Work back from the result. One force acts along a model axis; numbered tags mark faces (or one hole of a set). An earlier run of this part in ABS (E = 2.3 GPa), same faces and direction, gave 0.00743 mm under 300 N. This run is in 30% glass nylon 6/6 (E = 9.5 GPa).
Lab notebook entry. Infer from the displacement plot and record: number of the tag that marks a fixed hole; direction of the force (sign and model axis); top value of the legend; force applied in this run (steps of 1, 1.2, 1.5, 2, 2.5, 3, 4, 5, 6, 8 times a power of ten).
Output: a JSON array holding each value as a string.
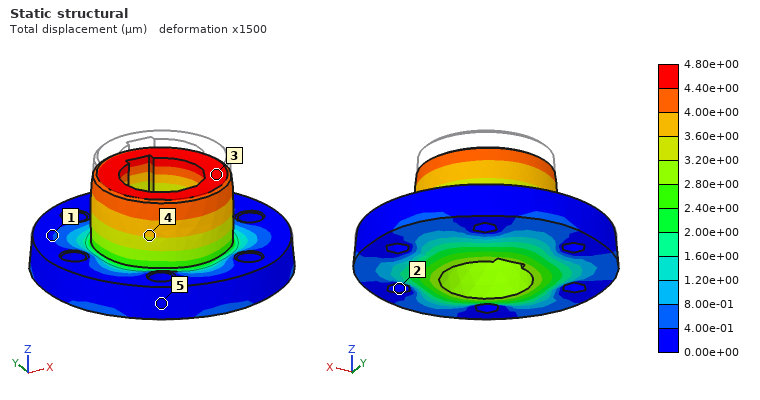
["2", "-Z", "4.80e+00 µm", "800 N"]
